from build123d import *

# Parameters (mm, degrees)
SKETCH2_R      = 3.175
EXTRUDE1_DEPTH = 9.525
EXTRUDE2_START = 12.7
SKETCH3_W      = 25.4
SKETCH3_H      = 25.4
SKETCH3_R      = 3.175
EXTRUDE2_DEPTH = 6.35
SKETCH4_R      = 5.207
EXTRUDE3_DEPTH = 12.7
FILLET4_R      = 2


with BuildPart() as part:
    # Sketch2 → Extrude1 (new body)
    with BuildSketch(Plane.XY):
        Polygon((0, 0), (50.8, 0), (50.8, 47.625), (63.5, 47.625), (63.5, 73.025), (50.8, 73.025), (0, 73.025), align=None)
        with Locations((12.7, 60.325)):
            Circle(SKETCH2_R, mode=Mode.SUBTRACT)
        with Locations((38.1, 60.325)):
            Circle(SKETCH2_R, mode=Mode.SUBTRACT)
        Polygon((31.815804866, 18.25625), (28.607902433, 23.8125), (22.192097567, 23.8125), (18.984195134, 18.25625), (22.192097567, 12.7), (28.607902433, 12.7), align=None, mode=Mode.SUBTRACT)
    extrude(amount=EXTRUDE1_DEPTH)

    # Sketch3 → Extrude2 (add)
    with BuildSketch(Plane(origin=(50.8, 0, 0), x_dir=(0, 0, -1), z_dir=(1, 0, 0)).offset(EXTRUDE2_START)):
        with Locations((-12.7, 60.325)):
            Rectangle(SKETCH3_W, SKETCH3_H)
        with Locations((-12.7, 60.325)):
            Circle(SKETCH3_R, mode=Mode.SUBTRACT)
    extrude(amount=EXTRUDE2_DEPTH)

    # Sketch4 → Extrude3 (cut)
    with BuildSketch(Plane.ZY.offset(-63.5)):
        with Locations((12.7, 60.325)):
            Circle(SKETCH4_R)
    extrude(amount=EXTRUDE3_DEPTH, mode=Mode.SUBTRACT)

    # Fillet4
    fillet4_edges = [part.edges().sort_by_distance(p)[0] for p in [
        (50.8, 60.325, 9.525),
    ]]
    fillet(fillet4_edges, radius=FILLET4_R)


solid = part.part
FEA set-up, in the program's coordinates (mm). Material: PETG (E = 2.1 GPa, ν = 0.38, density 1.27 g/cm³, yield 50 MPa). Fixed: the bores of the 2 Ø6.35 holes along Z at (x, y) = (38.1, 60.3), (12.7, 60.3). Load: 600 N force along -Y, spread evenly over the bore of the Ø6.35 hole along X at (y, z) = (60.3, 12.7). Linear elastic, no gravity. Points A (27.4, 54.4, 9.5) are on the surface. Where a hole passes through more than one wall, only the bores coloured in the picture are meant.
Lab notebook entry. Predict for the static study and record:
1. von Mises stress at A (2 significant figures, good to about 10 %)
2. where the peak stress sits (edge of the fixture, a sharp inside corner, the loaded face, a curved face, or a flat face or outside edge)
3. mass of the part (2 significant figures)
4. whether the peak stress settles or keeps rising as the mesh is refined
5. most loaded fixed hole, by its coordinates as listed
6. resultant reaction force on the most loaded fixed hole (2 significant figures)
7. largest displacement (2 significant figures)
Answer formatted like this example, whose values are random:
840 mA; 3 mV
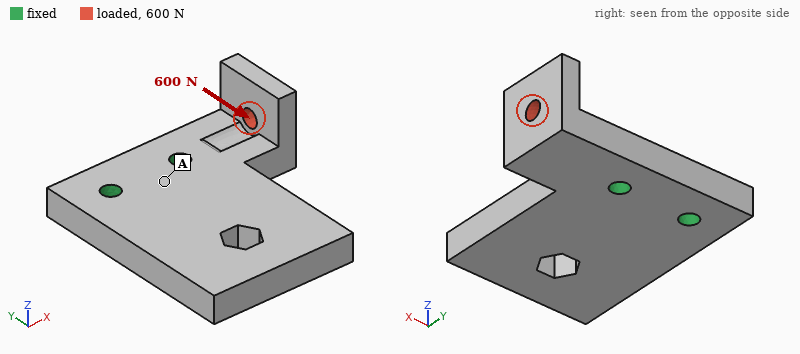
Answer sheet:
2.7 MPa; edge of the fixture; 51 g; keeps rising; (38.1, 60.3); 1.1 kN; 1.1 mm
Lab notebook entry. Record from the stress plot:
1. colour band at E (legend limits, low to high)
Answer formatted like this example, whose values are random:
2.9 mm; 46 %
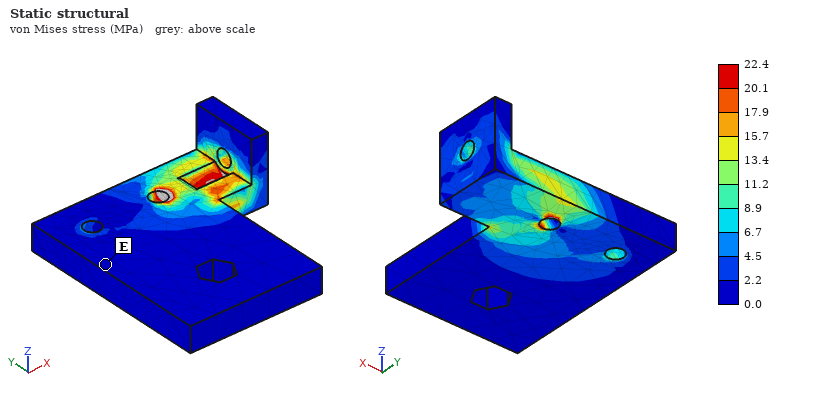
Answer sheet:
0.0 to 2.2 MPa
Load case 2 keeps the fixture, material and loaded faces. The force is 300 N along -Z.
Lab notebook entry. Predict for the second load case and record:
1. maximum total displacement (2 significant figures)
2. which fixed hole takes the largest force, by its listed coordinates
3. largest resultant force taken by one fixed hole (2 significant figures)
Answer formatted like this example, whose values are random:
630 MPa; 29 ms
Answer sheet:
0.94 mm; (38.1, 60.3); 400 N
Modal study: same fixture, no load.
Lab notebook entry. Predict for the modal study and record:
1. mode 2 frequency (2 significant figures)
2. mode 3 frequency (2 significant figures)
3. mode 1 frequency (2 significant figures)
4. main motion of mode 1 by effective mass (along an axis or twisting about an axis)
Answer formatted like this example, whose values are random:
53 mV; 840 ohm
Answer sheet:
1200 Hz; 1300 Hz; 560 Hz; along Z
